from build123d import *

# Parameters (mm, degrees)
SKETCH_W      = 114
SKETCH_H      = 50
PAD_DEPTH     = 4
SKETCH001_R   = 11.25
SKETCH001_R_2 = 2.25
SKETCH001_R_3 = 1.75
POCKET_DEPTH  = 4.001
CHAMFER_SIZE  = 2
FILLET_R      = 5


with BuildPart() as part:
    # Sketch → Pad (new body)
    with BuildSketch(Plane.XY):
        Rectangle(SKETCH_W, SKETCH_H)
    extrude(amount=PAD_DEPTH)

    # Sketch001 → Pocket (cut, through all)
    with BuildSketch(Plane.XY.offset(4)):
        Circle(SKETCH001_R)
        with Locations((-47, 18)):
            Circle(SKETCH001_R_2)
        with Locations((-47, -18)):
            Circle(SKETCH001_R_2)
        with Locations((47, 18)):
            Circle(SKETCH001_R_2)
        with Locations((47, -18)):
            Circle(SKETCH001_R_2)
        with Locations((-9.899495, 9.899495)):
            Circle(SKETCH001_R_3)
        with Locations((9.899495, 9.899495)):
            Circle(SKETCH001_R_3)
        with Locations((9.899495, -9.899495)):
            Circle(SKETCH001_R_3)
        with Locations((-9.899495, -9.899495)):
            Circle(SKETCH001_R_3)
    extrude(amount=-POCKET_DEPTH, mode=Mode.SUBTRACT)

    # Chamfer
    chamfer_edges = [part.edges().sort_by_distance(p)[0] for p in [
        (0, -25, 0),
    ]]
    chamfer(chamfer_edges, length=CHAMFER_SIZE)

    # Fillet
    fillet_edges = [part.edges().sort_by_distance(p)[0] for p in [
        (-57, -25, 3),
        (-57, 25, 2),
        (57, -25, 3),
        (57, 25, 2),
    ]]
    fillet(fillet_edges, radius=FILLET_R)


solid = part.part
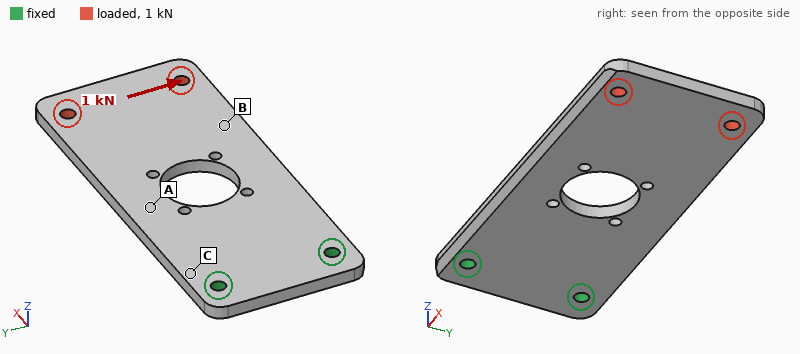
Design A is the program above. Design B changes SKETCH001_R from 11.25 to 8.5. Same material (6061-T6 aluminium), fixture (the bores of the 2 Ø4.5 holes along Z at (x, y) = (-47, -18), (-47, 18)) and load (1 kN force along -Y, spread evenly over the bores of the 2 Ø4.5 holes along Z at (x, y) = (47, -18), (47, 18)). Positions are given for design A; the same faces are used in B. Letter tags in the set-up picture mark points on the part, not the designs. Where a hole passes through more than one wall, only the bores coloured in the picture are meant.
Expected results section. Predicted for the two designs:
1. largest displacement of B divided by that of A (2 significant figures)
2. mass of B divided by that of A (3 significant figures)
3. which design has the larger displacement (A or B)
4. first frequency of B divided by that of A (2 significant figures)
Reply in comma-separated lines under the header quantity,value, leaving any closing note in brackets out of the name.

quantity,value
largest displacement of B divided by that of A,0.92
mass of B divided by that of A,1.03
which design has the larger displacement,A
first frequency of B divided by that of A,1.0
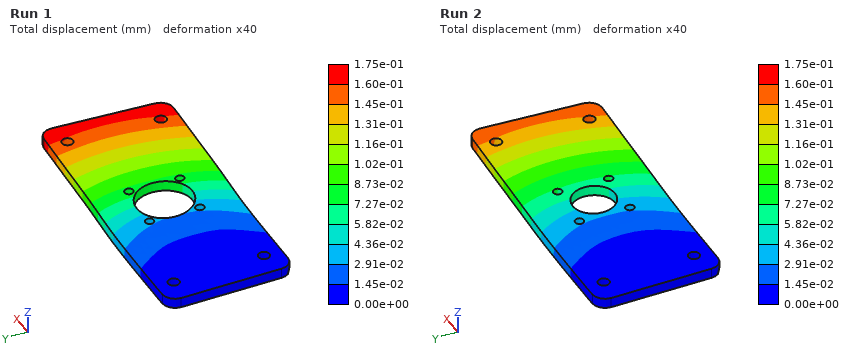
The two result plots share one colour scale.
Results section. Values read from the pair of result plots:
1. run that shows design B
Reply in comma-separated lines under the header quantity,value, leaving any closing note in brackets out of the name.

quantity,value
run that shows design B,Run 2
